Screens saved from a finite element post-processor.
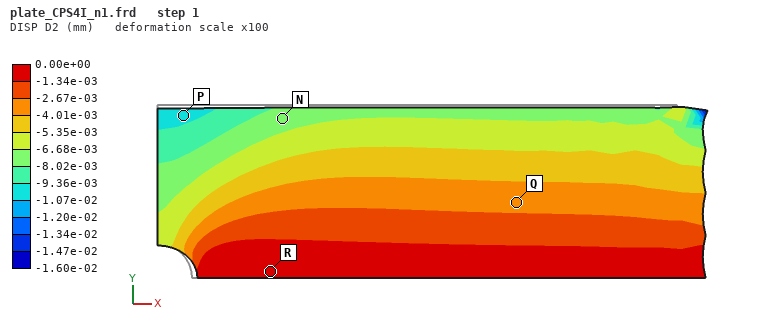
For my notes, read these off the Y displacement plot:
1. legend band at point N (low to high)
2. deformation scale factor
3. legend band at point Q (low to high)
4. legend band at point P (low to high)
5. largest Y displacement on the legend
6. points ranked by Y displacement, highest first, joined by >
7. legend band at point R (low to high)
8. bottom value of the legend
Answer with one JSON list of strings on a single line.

["-8.02e-03 to -6.68e-03 mm", "100", "-4.01e-03 to -2.67e-03 mm", "-1.07e-02 to -9.36e-03 mm", "0.00e+00 mm", "R > Q > N > P", "-1.34e-03 to 0.00e+00 mm", "-1.60e-02 mm"]
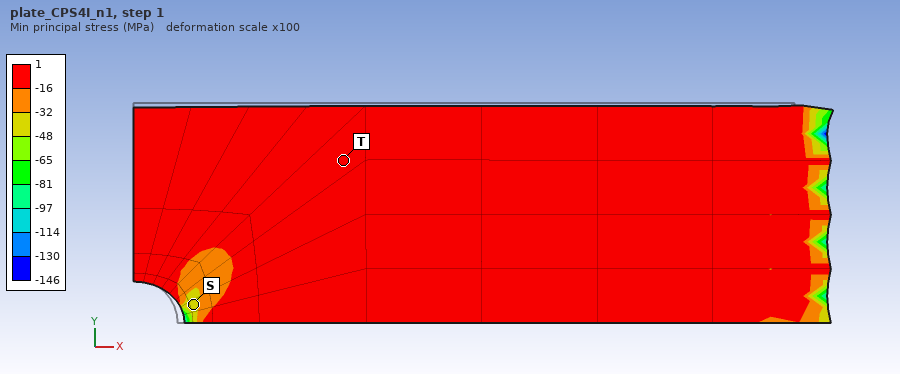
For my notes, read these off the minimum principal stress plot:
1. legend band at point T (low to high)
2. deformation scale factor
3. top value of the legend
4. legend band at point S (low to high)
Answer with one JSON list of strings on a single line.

["-16 to 1 MPa", "100", "1 MPa", "-48 to -32 MPa"]
